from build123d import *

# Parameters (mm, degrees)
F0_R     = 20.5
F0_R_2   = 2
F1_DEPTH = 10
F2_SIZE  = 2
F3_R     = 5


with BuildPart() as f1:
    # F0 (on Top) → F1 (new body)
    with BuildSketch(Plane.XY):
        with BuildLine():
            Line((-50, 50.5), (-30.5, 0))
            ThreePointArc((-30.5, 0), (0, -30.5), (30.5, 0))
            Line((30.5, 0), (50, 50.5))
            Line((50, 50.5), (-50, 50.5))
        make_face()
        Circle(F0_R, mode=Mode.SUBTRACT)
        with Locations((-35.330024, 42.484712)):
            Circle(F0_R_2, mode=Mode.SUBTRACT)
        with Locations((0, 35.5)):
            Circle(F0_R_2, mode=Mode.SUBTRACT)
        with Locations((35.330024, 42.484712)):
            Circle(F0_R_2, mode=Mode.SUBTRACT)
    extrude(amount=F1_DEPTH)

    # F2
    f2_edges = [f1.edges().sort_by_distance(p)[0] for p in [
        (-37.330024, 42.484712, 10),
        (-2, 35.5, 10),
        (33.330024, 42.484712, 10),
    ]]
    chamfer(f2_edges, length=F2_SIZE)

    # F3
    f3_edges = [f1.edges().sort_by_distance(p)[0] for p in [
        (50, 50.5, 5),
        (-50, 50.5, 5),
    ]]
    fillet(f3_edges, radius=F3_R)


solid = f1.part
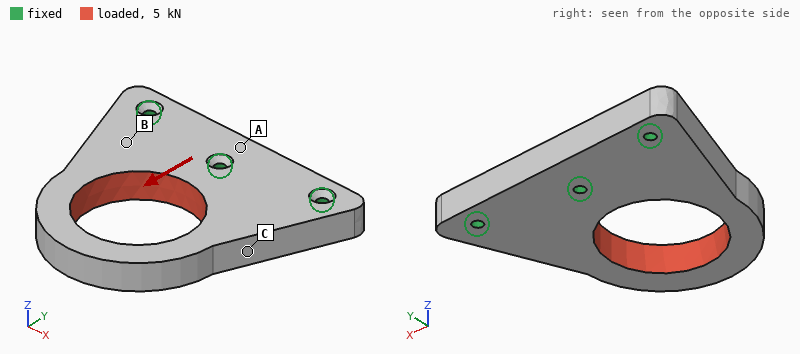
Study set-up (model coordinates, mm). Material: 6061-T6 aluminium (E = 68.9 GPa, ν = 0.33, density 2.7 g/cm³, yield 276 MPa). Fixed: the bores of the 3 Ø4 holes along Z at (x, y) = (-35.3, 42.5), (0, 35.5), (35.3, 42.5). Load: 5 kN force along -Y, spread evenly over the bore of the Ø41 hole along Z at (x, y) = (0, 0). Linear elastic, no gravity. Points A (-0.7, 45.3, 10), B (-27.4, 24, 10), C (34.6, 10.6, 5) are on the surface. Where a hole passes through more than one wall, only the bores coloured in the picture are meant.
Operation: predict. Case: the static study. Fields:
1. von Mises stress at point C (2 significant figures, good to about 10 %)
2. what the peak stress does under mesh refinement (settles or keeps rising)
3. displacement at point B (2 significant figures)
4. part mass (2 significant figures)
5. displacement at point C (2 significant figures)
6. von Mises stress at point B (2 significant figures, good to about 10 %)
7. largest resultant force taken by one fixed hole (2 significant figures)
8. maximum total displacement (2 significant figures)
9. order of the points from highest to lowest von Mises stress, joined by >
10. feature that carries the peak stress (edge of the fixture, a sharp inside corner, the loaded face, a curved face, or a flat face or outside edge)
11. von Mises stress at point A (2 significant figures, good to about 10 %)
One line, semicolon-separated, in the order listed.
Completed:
12 MPa; keeps rising; 3.7 µm; 110 g; 6.0 µm; 8.7 MPa; 1.7 kN; 20 µm; C > B > A; edge of the fixture; 3.0 MPa
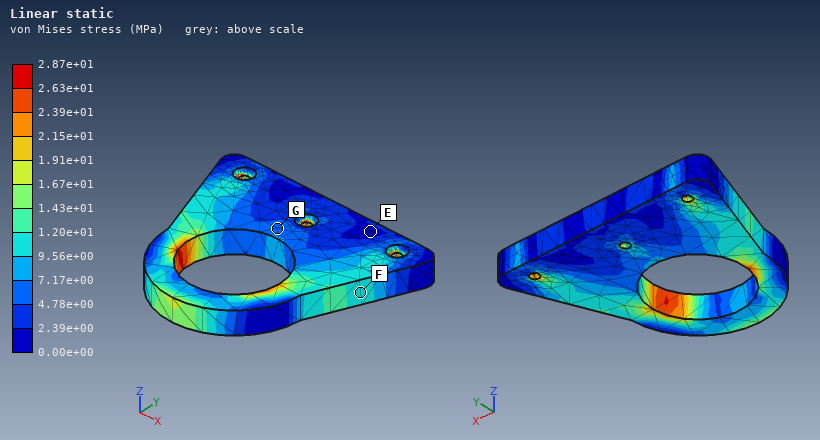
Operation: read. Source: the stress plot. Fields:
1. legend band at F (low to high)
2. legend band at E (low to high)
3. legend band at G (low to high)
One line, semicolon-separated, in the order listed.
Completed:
9.56e+00 to 1.20e+01 MPa; 0.00e+00 to 2.39e+00 MPa; 4.78e+00 to 7.17e+00 MPa
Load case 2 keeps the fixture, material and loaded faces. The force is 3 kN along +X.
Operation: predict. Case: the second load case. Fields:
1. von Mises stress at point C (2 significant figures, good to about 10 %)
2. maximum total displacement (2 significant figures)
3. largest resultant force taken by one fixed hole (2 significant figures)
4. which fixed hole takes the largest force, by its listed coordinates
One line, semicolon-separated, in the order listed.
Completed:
28 MPa; 46 µm; 1.9 kN; (0, 35.5)
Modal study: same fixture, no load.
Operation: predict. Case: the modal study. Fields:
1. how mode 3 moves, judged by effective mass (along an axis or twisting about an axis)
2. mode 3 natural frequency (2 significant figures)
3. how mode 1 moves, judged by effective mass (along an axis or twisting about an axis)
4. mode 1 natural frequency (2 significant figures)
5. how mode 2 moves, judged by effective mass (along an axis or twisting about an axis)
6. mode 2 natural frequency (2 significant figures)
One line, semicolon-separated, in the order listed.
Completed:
along X; 6800 Hz; along Z; 2000 Hz; twisting about Y; 4600 Hz
